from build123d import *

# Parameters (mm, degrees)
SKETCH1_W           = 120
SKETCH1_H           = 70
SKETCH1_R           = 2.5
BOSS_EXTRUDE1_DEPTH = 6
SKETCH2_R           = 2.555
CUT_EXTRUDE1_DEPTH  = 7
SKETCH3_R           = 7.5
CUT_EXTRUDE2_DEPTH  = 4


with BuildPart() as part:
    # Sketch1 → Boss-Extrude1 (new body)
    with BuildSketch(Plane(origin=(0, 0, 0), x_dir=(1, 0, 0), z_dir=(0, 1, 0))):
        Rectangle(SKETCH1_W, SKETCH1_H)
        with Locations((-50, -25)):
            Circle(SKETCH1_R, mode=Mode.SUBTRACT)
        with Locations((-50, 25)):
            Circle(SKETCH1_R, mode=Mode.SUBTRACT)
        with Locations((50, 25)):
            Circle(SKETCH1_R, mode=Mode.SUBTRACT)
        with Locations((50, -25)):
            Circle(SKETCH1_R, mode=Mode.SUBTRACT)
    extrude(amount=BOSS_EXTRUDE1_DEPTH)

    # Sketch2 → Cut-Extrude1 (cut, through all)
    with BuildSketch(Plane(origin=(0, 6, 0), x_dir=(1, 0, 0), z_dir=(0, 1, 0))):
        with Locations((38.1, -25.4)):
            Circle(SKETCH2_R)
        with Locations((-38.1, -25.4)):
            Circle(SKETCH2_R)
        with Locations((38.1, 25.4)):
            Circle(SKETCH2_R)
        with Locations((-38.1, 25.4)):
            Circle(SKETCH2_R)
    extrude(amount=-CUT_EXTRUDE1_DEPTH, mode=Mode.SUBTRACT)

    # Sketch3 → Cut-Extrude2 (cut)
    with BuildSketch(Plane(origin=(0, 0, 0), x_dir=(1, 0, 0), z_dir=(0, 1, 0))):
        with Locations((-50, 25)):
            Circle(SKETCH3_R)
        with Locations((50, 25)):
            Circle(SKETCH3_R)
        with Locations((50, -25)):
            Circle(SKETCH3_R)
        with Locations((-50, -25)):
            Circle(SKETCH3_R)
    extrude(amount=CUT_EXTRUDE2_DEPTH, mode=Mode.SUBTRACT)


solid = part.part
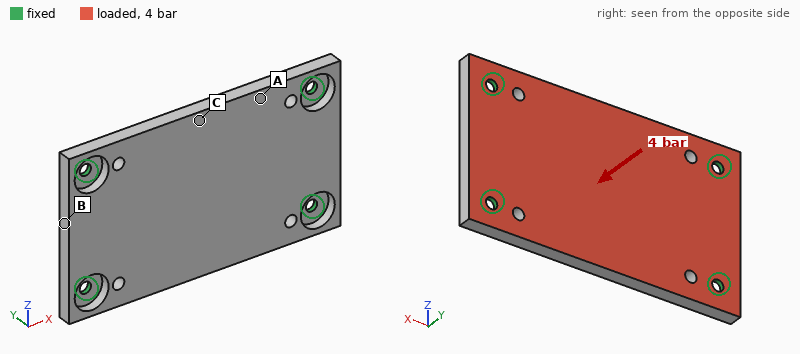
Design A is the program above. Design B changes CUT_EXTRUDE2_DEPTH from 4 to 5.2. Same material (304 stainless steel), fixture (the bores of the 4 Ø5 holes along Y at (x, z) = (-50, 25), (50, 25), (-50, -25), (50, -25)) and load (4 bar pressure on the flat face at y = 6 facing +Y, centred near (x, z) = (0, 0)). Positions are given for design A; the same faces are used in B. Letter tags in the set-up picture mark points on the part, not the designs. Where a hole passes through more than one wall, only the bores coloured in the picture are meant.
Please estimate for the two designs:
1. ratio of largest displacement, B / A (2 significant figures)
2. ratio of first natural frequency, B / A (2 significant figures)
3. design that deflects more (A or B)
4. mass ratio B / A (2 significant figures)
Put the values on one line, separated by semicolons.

1.7; 0.77; B; 0.98
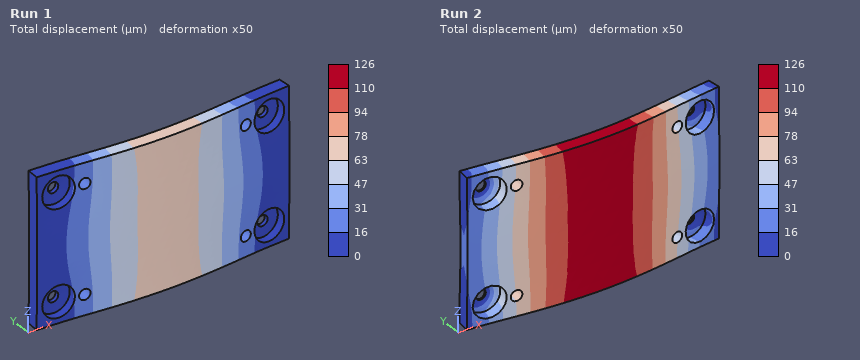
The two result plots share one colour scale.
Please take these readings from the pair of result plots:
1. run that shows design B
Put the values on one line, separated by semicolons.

Run 2
